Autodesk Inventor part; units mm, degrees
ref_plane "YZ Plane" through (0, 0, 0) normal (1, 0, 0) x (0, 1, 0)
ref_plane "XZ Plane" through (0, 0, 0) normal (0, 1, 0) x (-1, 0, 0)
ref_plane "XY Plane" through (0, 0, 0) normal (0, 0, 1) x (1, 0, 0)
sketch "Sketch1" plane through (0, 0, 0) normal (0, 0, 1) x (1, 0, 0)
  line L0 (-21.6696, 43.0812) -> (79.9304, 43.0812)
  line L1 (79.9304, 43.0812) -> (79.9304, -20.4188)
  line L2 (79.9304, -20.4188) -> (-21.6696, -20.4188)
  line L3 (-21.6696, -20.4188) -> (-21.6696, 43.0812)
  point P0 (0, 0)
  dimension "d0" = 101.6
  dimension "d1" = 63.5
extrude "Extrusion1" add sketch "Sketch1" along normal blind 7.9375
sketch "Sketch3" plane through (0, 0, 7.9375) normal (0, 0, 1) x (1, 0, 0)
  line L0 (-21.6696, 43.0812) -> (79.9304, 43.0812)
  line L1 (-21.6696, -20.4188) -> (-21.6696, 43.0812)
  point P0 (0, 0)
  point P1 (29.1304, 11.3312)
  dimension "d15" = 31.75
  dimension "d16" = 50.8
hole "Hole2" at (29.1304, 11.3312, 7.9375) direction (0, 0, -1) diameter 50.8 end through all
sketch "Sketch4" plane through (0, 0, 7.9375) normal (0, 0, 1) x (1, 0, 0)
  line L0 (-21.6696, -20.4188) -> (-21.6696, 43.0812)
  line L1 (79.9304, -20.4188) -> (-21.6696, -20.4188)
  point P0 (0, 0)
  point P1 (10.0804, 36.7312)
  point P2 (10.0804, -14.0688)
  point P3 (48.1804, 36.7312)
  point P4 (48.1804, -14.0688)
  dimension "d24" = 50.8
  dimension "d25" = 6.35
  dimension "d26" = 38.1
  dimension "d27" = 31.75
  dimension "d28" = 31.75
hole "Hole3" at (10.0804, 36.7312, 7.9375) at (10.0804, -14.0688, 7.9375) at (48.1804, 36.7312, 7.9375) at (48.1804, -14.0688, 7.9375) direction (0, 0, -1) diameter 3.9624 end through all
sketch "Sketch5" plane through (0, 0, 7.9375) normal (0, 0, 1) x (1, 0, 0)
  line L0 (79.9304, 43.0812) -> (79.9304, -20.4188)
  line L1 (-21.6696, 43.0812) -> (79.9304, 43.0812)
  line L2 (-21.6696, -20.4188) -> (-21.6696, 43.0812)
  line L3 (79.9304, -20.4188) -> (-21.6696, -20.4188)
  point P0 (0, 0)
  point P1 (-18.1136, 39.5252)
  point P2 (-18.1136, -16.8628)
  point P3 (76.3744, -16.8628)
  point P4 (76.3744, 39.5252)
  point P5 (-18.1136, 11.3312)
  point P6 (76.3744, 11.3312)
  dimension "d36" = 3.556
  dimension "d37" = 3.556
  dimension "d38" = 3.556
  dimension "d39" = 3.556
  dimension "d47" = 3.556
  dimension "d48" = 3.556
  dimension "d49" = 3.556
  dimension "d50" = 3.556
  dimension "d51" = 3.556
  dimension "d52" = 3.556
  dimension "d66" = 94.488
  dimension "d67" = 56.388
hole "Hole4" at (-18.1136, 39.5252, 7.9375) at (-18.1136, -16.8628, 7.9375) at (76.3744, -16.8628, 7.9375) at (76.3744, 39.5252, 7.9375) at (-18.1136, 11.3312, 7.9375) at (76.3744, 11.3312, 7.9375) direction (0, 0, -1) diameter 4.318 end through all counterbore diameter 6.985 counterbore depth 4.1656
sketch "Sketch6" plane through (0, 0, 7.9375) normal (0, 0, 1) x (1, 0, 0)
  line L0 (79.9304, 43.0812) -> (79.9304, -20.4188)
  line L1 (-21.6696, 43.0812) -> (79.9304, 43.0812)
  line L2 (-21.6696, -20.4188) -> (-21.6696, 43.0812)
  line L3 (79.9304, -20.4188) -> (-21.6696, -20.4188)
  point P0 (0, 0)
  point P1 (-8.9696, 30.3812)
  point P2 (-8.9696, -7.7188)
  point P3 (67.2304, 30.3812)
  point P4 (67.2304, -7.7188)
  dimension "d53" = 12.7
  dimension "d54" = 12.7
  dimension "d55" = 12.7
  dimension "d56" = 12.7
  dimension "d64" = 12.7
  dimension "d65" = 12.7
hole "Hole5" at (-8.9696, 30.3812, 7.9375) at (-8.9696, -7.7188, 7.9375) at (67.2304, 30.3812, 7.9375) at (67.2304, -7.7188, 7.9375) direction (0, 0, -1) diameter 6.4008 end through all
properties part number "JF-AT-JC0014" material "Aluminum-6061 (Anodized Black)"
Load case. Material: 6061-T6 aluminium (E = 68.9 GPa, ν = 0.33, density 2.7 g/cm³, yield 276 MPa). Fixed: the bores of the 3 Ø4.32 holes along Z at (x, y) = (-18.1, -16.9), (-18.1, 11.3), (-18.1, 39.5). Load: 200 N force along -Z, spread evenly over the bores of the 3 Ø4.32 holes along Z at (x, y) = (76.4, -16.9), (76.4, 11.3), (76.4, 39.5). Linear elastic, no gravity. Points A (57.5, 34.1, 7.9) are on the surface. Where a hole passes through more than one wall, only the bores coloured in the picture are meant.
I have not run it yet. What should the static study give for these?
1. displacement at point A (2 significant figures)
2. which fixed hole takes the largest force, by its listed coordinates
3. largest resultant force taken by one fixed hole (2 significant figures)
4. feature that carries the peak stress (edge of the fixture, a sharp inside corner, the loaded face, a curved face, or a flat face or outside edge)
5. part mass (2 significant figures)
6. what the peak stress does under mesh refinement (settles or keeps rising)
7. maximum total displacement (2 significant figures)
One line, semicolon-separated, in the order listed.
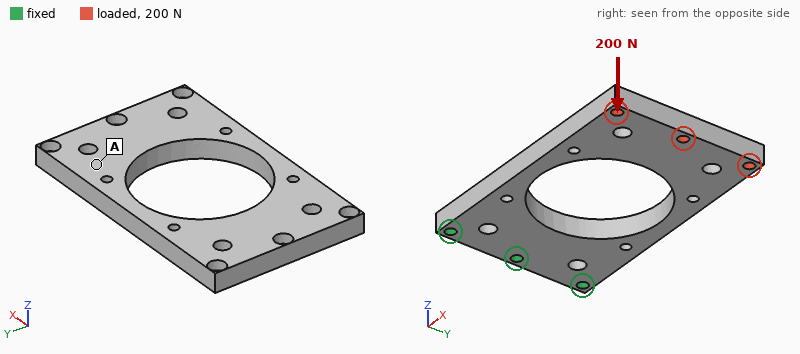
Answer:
0.69 mm; (-18.1, 11.3); 220 N; edge of the fixture; 88 g; keeps rising; 1.0 mm
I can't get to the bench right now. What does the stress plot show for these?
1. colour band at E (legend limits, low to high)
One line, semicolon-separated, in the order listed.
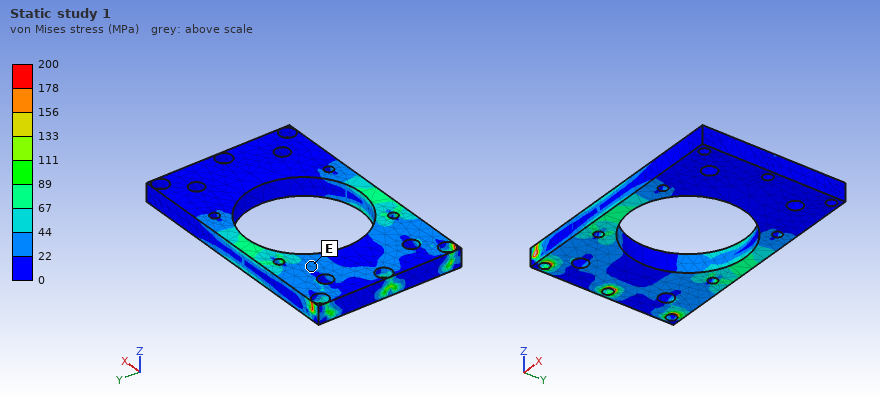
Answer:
22 to 44 MPa
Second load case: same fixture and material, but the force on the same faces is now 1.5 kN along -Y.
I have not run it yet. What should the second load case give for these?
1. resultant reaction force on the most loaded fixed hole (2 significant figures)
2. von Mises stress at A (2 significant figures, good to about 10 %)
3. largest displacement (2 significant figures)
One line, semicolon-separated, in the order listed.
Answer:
2.5 kN; 14 MPa; 0.28 mm
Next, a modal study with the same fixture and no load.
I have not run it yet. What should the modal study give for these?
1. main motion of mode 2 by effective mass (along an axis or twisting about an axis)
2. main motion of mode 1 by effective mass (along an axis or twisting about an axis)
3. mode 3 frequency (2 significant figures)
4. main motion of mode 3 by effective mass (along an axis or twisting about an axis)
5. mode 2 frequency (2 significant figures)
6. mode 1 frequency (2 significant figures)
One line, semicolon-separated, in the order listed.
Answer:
twisting about X; along Z; 2100 Hz; along Y; 1500 Hz; 440 Hz
